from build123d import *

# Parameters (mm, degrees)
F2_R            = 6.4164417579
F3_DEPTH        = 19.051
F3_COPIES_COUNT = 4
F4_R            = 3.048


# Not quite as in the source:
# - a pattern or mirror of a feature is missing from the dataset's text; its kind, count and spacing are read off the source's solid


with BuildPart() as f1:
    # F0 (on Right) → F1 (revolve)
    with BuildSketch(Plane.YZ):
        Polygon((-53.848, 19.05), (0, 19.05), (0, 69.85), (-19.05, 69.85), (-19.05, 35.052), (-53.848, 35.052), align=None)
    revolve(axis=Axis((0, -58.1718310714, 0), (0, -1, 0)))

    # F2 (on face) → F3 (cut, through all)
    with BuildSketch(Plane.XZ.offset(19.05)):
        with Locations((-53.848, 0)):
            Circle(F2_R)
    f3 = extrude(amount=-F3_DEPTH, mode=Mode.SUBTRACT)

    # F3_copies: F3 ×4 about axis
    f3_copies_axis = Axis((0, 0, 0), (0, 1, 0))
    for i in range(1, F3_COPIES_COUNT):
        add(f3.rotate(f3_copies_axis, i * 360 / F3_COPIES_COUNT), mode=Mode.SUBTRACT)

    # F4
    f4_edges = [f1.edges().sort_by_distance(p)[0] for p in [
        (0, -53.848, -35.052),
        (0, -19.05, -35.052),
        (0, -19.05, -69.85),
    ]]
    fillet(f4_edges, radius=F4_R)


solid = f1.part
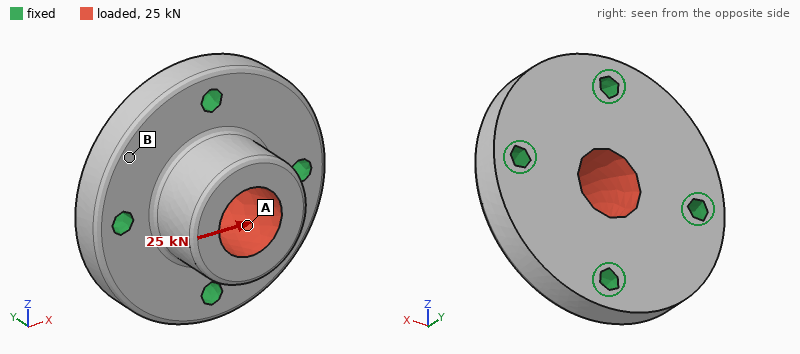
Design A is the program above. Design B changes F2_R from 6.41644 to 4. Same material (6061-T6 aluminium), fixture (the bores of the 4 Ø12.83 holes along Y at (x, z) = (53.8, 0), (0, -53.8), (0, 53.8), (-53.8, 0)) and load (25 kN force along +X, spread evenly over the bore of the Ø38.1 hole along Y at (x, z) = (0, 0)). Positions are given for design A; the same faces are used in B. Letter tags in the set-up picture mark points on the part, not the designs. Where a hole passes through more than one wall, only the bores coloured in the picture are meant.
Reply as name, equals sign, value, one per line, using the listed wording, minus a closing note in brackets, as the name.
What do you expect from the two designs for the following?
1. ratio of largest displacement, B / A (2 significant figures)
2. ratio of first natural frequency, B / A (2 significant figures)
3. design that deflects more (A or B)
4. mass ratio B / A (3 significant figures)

ratio of largest displacement, B / A = 1.1
ratio of first natural frequency, B / A = 0.90
design that deflects more = B
mass ratio B / A = 1.02
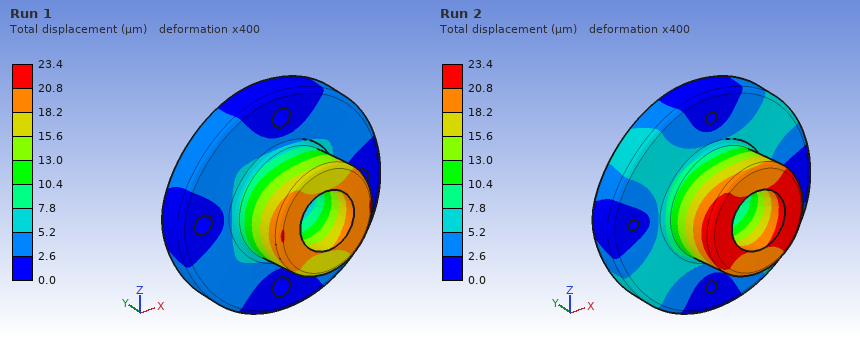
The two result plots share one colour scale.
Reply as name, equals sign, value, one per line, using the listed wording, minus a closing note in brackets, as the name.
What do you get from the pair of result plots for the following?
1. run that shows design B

run that shows design B = Run 2
